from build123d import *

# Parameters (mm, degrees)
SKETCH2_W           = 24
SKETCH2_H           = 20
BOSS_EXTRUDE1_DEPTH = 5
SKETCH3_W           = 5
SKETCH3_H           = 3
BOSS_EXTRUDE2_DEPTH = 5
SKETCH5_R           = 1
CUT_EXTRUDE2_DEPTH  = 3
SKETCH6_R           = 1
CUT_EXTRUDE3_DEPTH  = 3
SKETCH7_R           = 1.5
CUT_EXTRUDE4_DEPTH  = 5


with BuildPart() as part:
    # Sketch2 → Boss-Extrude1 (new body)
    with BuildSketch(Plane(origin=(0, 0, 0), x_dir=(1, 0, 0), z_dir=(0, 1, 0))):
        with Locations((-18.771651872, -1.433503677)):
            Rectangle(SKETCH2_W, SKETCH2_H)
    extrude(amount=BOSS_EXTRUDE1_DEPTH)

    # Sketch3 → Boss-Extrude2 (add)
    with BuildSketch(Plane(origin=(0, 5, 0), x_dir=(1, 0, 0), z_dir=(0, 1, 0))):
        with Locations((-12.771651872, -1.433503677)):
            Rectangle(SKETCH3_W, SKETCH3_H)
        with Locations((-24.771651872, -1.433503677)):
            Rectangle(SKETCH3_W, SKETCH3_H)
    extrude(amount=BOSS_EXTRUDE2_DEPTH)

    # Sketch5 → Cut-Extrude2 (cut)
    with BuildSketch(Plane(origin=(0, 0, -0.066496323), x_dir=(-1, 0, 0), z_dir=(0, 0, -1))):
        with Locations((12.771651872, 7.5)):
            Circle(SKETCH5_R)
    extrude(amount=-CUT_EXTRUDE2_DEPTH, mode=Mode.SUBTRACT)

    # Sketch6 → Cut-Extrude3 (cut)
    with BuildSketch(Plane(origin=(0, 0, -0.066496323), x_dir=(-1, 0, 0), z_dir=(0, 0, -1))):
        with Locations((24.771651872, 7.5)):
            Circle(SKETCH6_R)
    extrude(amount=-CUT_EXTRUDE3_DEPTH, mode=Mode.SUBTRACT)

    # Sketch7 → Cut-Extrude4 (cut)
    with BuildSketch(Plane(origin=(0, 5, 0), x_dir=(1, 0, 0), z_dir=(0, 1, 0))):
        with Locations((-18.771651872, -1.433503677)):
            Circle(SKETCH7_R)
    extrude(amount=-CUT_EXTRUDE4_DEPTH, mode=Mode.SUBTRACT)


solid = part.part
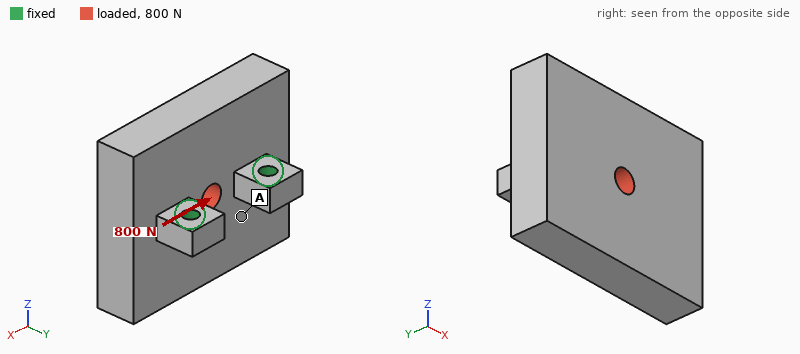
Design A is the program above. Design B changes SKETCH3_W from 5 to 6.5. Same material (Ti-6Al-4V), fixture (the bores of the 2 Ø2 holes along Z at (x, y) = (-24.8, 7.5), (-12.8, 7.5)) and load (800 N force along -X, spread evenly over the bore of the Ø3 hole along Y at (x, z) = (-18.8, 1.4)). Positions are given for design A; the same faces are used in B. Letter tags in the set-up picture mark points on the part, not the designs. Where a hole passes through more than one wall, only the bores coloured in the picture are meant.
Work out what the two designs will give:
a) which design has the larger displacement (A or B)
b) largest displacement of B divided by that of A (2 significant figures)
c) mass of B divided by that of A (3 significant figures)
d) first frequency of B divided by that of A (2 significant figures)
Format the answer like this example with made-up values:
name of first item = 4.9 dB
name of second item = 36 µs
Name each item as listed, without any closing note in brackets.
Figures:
which design has the larger displacement = A
largest displacement of B divided by that of A = 0.89
mass of B divided by that of A = 1.02
first frequency of B divided by that of A = 1.1
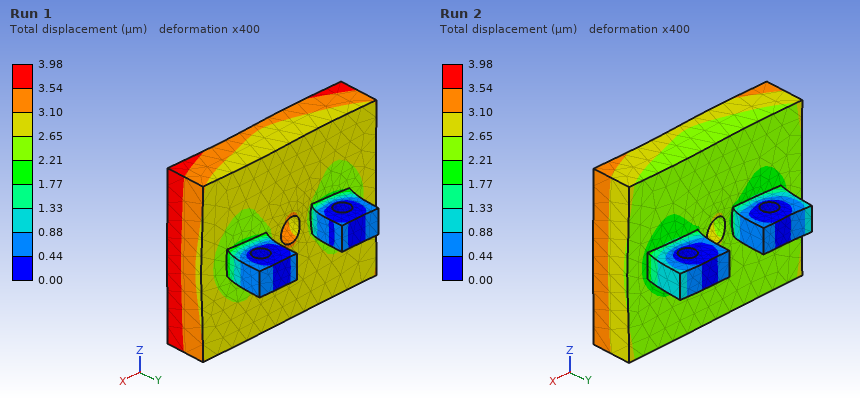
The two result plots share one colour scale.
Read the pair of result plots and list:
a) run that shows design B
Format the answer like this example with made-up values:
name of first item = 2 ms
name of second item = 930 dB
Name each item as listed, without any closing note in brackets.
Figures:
run that shows design B = Run 2
